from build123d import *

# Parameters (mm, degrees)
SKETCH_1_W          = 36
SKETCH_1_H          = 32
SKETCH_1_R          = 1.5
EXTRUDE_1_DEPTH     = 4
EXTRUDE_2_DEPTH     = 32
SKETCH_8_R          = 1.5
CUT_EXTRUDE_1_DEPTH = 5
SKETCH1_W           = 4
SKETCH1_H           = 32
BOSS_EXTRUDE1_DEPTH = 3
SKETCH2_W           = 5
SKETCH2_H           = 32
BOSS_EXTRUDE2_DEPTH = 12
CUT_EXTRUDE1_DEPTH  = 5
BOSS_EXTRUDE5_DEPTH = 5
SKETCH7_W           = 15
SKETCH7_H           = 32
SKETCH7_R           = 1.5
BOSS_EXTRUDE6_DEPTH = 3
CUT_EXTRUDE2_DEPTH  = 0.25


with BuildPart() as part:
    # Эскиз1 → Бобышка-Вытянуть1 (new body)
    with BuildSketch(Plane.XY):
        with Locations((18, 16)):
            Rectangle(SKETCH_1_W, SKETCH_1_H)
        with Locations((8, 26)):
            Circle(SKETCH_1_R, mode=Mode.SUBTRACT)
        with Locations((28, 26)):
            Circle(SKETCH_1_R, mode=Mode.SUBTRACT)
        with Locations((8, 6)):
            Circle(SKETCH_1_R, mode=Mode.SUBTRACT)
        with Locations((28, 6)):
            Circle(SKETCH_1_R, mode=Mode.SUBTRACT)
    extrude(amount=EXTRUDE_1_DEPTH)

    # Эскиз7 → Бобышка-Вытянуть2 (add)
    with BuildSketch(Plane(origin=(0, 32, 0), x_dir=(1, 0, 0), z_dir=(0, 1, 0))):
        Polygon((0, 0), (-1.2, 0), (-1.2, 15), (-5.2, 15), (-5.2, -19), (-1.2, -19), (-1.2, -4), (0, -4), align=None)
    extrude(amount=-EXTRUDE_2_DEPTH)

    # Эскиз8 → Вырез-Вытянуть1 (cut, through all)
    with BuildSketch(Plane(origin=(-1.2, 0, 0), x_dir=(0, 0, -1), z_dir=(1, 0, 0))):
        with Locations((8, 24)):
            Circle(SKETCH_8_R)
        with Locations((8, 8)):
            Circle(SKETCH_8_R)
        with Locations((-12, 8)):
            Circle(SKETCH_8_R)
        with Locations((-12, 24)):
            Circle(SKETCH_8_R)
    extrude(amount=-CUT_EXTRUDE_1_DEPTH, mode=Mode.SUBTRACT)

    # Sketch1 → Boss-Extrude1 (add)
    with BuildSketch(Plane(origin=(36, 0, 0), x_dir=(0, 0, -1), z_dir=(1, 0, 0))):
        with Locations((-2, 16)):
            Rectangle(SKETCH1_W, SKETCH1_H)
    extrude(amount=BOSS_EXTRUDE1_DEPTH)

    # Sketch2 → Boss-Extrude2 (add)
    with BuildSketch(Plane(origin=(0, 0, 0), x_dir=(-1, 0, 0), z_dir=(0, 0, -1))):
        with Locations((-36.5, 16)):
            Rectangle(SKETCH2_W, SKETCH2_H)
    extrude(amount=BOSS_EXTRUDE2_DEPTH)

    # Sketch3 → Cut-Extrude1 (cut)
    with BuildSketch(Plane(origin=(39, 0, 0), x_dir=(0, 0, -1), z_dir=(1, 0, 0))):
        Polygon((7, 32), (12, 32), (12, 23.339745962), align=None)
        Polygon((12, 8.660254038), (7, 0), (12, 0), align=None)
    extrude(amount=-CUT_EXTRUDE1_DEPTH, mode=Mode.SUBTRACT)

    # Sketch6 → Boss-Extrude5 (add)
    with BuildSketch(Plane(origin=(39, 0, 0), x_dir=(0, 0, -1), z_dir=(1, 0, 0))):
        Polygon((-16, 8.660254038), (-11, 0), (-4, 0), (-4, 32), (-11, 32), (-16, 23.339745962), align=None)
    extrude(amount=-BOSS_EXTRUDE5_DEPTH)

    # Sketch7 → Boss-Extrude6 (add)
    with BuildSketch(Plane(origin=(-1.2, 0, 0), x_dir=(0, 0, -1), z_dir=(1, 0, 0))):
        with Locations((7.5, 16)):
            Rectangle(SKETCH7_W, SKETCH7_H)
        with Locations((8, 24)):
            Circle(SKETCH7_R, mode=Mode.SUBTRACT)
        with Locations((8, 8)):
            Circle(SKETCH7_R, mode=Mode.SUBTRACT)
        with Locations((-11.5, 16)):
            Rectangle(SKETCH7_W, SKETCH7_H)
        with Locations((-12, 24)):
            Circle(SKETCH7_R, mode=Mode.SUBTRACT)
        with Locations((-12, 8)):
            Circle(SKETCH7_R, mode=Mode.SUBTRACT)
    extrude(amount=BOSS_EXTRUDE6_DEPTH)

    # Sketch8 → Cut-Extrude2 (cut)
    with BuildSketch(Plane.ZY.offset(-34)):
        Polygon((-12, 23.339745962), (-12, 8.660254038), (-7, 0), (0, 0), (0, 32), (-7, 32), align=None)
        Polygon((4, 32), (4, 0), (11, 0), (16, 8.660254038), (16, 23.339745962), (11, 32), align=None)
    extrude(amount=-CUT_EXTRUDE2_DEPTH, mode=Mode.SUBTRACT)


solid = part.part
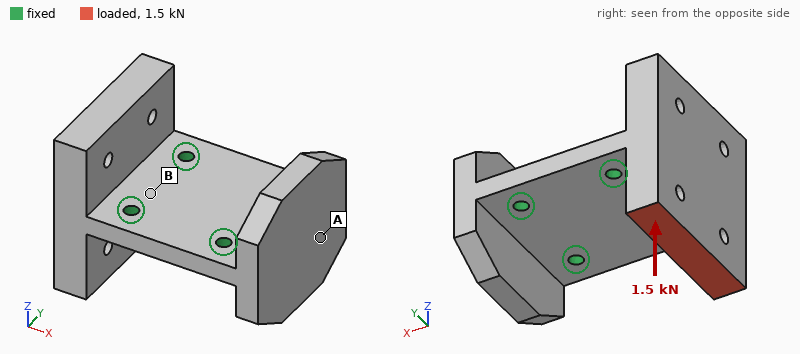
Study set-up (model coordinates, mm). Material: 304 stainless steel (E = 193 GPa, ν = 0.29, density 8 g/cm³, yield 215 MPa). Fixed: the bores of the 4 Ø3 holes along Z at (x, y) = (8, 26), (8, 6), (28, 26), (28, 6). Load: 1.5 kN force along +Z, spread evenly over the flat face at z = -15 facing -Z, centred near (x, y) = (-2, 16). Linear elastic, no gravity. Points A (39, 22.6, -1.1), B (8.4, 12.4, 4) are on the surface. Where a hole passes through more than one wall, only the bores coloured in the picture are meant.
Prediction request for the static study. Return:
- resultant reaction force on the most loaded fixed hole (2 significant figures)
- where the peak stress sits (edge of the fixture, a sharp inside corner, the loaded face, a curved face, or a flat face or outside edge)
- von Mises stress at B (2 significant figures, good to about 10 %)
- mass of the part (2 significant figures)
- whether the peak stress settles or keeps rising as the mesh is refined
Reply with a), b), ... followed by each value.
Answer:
a) 840 N
b) edge of the fixture
c) 60 MPa
d) 120 g
e) keeps rising
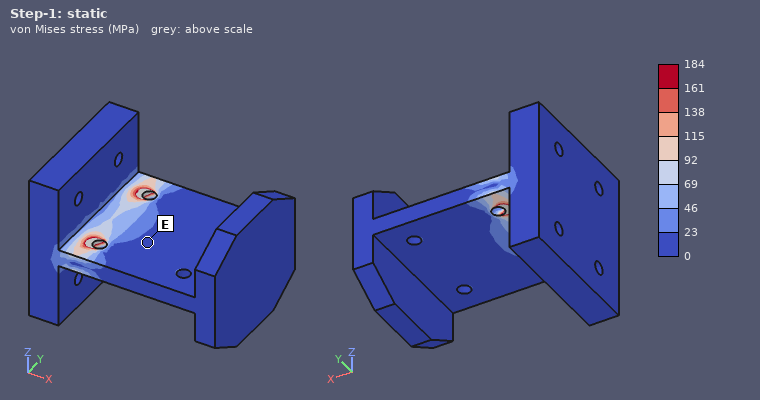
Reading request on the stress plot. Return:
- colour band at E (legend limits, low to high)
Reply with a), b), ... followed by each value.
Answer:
a) 0 to 23 MPa
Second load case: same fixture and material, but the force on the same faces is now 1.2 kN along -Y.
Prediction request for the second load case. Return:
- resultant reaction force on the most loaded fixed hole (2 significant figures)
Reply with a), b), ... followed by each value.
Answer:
a) 1.2 kN
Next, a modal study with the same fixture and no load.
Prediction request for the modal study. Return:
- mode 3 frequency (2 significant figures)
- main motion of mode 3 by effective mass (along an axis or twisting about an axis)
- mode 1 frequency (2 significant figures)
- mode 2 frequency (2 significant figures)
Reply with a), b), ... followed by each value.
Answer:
a) 9100 Hz
b) twisting about X
c) 3600 Hz
d) 6300 Hz
